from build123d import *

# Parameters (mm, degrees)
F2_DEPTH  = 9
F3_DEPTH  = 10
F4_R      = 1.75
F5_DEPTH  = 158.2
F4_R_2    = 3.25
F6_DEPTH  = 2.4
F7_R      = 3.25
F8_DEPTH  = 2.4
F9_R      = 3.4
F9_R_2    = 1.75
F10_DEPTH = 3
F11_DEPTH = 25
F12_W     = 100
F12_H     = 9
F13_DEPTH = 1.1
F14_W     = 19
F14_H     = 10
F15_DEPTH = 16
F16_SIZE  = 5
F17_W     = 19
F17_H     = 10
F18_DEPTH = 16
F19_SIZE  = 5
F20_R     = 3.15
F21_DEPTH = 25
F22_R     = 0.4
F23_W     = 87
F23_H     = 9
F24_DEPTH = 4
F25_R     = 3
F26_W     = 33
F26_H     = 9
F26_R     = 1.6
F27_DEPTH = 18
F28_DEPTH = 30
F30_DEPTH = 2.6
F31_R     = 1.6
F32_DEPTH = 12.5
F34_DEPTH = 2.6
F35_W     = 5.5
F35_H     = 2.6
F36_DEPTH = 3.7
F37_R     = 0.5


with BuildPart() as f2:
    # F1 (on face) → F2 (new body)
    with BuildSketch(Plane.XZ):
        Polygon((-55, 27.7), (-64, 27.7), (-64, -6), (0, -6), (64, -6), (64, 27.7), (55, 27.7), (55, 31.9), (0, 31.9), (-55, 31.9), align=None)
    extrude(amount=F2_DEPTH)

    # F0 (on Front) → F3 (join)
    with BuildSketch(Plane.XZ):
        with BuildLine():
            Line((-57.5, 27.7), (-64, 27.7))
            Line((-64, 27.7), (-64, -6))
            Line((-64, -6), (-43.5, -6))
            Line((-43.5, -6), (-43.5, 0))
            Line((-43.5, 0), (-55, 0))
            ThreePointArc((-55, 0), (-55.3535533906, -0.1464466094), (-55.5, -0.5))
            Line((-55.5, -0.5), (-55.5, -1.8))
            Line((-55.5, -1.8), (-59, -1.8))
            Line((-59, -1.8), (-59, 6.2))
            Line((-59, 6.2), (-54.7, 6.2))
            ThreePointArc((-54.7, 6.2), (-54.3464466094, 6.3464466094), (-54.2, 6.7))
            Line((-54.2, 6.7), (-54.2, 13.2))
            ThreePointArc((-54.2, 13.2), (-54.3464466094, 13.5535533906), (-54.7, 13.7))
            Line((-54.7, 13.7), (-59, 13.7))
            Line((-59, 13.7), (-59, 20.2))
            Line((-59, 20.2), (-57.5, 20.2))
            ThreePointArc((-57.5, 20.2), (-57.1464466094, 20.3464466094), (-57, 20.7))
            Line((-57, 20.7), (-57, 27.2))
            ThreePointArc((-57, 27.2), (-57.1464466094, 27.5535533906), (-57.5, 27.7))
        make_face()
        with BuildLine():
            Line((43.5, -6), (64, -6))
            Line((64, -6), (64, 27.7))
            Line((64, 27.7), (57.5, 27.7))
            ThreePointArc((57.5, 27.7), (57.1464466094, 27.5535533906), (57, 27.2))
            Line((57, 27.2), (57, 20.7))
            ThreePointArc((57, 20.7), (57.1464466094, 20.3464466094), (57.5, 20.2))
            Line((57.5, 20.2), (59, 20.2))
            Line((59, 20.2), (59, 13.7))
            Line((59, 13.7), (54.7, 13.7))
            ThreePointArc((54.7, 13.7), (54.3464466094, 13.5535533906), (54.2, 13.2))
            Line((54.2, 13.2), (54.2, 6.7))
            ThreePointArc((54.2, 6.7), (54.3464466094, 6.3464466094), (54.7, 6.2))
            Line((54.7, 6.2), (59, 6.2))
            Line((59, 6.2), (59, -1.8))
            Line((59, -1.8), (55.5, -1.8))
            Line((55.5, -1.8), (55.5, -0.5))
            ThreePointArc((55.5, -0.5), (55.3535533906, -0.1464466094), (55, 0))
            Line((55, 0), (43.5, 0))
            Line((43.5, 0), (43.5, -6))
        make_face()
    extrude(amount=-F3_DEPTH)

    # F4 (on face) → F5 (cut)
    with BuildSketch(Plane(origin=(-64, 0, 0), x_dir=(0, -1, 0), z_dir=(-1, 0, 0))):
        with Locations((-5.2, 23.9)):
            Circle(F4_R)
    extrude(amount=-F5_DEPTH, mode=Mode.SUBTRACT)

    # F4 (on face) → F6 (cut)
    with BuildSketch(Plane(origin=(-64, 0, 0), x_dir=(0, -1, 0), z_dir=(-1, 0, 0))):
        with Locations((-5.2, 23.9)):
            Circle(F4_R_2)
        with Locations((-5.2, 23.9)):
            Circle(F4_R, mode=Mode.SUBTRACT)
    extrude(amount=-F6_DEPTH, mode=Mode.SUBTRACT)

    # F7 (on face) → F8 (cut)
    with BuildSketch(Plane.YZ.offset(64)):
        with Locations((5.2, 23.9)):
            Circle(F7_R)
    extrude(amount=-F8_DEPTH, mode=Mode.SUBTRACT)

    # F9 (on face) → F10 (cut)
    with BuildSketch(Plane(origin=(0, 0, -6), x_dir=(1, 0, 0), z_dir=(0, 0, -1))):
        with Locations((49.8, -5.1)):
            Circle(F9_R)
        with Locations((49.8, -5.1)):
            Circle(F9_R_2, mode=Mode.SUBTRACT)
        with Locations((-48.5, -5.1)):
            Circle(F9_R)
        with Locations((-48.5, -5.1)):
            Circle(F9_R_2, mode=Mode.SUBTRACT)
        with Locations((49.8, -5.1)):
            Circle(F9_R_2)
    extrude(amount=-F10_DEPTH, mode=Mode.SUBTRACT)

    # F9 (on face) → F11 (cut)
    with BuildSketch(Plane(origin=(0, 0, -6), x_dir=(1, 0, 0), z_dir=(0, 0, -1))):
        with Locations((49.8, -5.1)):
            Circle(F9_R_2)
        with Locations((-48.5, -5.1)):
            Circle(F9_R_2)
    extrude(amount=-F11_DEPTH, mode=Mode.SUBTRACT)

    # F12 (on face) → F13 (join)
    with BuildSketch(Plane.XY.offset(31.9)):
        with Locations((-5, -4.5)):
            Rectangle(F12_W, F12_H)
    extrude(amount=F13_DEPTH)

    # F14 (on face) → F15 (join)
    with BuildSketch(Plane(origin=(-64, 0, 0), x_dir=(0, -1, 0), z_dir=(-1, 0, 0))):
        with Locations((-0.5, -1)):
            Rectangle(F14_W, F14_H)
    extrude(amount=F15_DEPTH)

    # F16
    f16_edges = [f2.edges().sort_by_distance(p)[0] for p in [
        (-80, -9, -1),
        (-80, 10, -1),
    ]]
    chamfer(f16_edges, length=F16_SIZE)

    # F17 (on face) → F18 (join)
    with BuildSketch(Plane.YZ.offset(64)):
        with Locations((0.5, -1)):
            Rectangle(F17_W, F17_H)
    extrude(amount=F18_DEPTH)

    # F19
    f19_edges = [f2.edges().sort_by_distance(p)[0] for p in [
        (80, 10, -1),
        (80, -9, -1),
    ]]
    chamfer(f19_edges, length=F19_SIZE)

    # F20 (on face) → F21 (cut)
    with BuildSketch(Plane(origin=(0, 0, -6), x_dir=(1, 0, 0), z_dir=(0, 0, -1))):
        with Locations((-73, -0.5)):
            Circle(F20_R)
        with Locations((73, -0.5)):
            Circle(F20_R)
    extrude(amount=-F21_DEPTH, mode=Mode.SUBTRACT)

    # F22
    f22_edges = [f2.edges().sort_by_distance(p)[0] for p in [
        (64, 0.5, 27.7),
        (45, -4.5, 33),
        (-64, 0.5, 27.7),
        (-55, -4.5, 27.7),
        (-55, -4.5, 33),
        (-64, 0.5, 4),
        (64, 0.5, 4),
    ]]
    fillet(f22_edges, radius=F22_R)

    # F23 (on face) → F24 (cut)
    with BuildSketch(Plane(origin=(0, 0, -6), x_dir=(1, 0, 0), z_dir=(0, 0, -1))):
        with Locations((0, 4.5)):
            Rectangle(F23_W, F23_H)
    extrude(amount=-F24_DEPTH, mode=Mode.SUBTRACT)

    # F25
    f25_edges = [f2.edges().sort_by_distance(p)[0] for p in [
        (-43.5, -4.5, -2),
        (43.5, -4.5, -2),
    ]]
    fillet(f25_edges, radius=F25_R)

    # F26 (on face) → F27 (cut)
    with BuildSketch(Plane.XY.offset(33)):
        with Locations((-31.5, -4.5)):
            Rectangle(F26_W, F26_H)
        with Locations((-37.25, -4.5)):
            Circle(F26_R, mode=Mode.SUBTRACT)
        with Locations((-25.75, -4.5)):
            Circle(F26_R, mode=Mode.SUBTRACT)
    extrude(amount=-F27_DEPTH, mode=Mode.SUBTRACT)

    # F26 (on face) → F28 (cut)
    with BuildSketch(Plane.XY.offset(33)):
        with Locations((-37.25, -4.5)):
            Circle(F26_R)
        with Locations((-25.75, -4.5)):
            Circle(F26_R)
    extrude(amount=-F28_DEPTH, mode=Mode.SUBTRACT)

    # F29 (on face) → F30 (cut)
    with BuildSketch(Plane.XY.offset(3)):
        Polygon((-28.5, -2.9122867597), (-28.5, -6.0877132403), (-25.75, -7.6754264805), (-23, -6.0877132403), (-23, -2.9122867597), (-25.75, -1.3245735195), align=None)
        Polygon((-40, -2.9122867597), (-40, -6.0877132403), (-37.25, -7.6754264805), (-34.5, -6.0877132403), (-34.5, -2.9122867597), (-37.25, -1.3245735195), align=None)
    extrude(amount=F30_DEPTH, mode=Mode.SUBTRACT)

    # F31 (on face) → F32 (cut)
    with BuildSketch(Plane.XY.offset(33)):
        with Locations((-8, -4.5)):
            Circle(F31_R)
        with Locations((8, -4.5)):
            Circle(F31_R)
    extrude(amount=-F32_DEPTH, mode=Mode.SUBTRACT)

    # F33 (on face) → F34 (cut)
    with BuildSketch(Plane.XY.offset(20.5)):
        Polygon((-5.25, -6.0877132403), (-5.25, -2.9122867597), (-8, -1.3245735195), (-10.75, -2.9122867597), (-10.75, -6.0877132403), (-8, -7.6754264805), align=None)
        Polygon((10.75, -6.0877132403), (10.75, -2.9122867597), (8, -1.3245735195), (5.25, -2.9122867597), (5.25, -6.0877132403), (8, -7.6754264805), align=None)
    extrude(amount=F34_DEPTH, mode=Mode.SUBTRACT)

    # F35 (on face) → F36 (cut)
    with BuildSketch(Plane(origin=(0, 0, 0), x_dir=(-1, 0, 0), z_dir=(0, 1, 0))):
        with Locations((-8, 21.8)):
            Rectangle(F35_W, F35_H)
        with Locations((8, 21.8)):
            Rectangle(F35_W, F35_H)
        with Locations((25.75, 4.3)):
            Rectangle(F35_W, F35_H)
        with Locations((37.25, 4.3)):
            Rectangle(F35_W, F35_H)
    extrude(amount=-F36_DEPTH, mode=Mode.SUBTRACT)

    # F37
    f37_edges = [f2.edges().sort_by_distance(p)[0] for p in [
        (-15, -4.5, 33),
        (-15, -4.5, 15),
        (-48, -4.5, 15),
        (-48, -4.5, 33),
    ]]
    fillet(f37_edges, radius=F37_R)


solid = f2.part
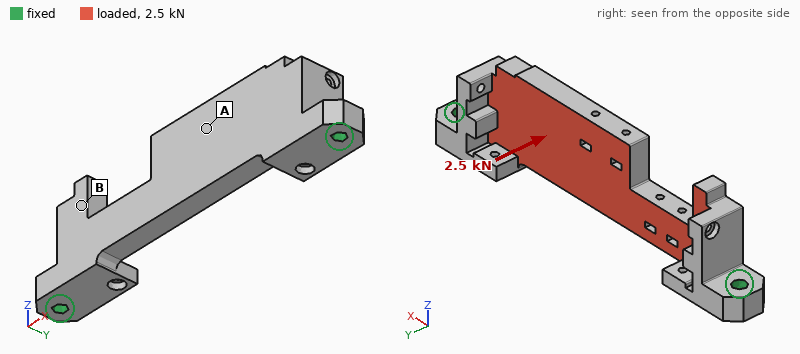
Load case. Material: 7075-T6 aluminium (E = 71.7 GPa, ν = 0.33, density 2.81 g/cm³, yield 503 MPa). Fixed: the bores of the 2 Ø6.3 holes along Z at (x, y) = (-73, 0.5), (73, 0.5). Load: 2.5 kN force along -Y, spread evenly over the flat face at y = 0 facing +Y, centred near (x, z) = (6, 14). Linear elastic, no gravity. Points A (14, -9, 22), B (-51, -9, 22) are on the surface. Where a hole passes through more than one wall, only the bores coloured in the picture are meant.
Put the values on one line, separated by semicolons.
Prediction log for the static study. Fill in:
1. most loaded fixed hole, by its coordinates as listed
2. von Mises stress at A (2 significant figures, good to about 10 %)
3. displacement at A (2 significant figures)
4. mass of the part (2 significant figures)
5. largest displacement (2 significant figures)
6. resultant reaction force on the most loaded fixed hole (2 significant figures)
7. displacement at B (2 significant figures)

(73, 0.5); 31 MPa; 0.23 mm; 130 g; 0.30 mm; 1.6 kN; 0.070 mm
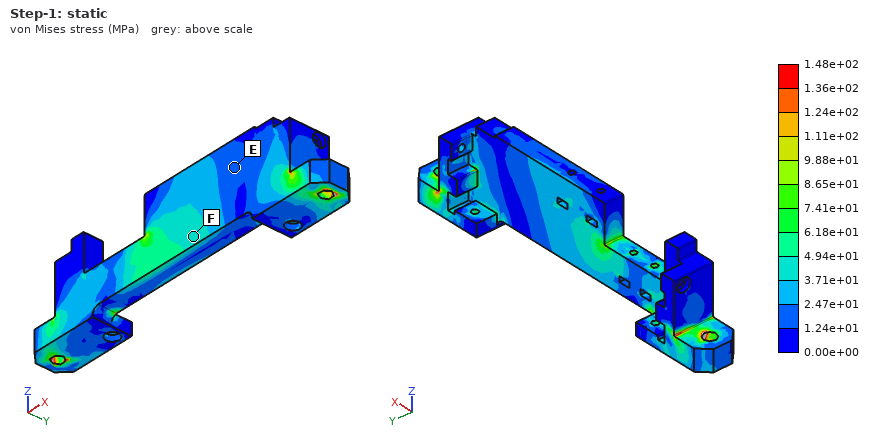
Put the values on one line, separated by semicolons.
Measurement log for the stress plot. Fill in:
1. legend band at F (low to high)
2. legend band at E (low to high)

3.71e+01 to 4.94e+01 MPa; 1.24e+01 to 2.47e+01 MPa
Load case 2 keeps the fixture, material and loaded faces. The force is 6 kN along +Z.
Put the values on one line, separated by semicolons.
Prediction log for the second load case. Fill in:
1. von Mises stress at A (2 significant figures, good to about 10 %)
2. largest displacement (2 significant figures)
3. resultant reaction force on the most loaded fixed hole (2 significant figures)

24 MPa; 0.21 mm; 4.9 kN
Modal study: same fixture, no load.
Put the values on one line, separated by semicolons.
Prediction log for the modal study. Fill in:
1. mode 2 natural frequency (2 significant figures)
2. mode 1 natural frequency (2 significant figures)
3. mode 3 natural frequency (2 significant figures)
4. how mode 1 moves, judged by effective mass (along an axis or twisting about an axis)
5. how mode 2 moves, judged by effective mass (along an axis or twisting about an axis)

3500 Hz; 2000 Hz; 4400 Hz; along Y; along Z
